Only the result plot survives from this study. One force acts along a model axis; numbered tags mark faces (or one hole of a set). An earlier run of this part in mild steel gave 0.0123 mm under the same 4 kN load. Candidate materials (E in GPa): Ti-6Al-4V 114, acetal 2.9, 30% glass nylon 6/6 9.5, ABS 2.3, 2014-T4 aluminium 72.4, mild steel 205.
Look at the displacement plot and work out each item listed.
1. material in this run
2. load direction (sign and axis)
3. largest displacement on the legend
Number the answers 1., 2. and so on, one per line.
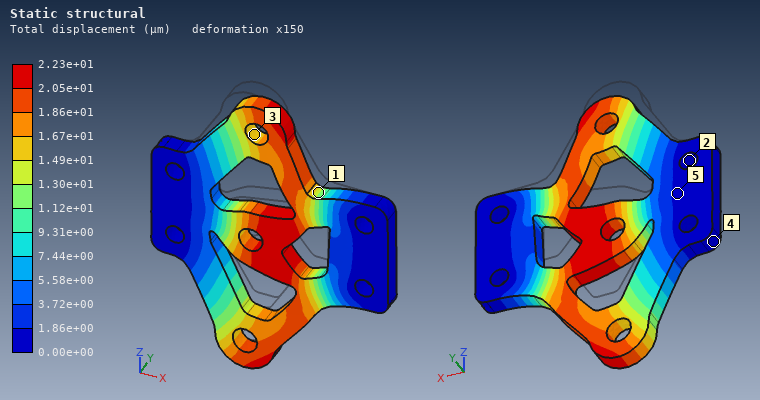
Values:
1. Ti-6Al-4V
2. -Z
3. 2.23e+01 µm
